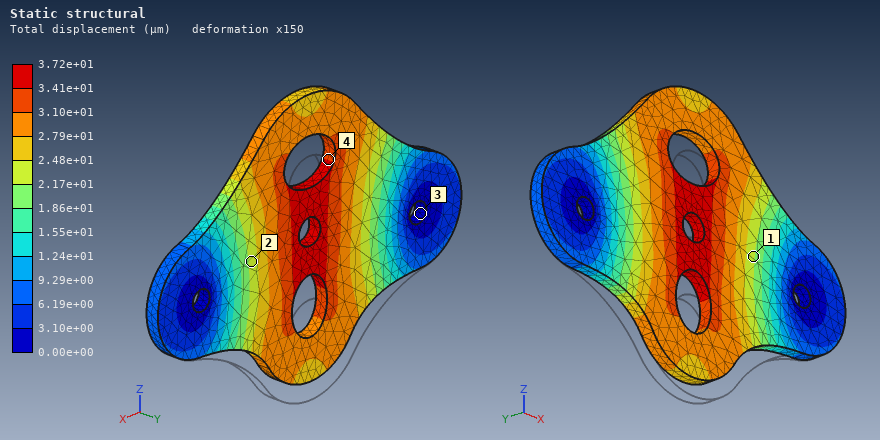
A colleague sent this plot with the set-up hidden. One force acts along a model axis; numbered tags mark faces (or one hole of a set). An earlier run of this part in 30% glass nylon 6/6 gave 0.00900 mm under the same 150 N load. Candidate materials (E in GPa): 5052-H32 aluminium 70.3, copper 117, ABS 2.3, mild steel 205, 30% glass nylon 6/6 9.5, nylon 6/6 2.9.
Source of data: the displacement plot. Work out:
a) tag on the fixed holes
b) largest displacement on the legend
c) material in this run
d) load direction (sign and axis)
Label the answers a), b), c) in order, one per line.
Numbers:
a) 3
b) 3.72e+01 µm
c) ABS
d) +Z
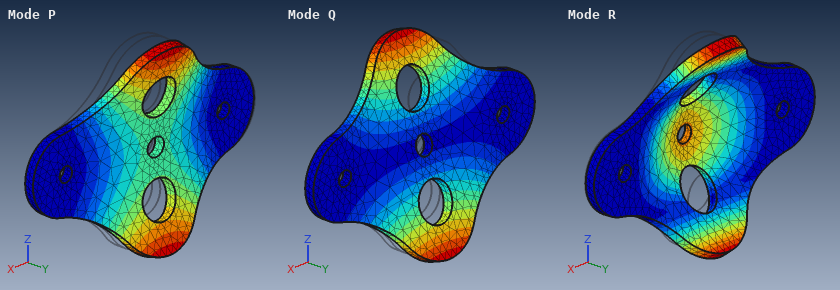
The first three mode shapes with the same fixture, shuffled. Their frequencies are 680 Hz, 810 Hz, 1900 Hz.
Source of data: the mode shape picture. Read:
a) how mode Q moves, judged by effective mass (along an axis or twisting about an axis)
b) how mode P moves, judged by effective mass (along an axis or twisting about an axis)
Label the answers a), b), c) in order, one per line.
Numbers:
a) twisting about X
b) along Y
